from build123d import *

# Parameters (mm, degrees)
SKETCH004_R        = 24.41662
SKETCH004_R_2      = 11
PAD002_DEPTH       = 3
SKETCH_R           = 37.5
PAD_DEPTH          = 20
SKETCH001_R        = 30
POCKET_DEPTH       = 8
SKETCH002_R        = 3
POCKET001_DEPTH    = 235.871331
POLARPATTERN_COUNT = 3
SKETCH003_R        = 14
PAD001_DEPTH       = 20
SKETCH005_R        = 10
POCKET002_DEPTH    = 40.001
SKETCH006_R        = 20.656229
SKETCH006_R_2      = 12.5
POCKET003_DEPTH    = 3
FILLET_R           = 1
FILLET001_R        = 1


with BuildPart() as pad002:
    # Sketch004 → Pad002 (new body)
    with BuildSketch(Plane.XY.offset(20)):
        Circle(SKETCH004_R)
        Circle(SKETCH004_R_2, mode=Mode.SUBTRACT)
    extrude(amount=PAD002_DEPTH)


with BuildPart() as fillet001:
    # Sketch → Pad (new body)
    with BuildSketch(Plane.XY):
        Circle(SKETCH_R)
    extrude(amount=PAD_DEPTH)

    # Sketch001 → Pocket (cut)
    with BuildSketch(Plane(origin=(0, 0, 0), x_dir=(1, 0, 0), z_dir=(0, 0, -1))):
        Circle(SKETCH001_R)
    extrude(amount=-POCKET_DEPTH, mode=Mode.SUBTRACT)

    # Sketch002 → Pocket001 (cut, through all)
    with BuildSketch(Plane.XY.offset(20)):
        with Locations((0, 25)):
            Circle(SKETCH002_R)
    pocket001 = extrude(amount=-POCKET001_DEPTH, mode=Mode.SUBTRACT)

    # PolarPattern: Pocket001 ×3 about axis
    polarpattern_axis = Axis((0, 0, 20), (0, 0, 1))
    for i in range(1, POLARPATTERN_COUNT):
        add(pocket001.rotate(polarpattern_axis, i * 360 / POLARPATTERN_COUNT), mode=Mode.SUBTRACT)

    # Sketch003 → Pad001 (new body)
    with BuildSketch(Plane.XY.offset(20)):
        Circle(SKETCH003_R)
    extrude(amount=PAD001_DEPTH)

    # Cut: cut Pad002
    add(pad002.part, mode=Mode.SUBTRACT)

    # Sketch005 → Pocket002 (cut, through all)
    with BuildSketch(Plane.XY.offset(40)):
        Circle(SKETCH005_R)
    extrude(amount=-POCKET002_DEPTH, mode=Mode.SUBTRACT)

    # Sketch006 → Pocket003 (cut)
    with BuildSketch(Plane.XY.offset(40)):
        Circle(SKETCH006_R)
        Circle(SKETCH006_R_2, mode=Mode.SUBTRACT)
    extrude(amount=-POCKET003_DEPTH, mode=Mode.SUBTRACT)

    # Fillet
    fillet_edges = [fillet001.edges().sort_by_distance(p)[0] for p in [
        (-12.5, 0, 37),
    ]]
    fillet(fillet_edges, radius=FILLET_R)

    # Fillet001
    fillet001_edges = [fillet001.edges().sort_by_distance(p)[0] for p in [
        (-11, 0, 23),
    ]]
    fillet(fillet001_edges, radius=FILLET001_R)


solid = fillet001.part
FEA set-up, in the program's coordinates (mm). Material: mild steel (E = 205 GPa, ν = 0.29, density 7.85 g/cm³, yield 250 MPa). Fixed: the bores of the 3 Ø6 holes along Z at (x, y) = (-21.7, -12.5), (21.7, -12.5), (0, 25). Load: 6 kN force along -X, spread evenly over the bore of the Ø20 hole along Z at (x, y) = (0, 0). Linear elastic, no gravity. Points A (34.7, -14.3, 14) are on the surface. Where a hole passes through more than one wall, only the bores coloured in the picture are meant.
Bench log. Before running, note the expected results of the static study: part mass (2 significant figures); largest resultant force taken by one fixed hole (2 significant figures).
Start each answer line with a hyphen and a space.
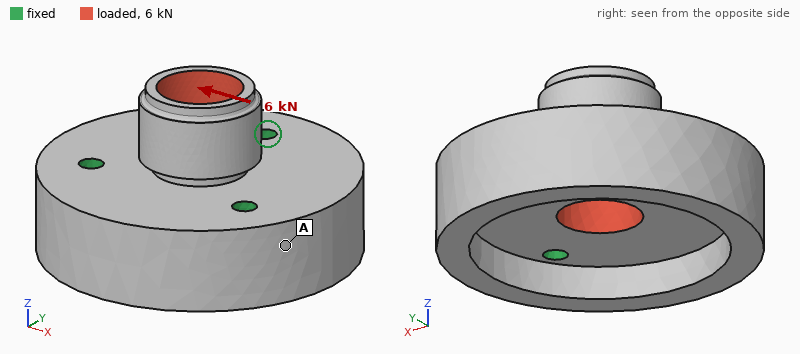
- 520 g
- 2.4 kN
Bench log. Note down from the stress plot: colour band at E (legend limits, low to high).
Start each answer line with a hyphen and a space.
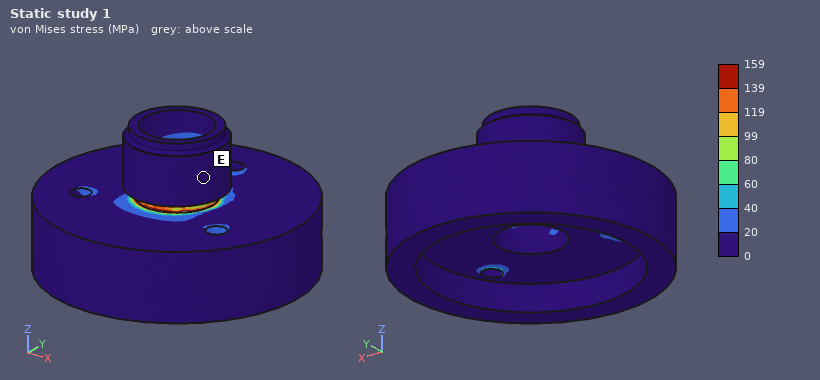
- 0 to 20 MPa
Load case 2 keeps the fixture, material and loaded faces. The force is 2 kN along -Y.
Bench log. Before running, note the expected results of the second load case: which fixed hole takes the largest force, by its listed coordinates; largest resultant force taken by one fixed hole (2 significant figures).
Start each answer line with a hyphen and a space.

- (0, 25)
- 850 N
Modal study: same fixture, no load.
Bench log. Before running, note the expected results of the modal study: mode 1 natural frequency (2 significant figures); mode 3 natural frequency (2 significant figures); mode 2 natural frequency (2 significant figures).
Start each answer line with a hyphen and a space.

- 11 kHz
- 12 kHz
- 11 kHz
